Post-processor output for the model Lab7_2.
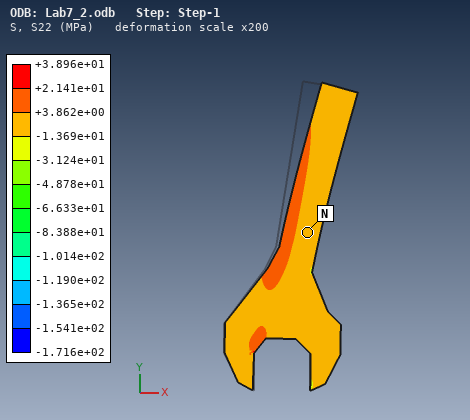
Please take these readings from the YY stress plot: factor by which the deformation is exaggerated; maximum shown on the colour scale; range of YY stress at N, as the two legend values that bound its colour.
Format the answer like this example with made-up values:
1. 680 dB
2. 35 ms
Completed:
1. 200
2. +3.896e+01 MPa
3. -1.369e+01 to +3.862e+00 MPa
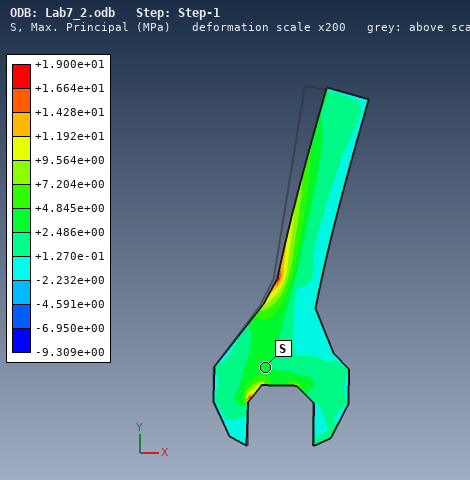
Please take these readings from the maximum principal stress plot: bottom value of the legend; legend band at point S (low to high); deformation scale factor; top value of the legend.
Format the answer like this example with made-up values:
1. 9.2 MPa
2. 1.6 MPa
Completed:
1. -9.309e+00 MPa
2. +2.486e+00 to +4.845e+00 MPa
3. 200
4. +1.900e+01 MPa
